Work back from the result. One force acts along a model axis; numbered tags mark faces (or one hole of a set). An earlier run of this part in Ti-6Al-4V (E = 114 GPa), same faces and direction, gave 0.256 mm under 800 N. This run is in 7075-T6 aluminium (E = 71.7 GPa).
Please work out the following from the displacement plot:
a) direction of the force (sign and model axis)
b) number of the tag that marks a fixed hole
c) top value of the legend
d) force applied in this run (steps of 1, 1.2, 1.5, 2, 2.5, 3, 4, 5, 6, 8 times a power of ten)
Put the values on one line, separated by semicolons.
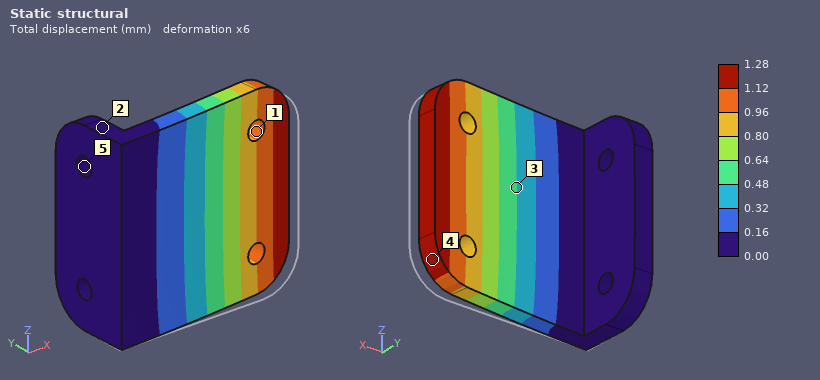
+Y; 5; 1.28 mm; 2.5 kN
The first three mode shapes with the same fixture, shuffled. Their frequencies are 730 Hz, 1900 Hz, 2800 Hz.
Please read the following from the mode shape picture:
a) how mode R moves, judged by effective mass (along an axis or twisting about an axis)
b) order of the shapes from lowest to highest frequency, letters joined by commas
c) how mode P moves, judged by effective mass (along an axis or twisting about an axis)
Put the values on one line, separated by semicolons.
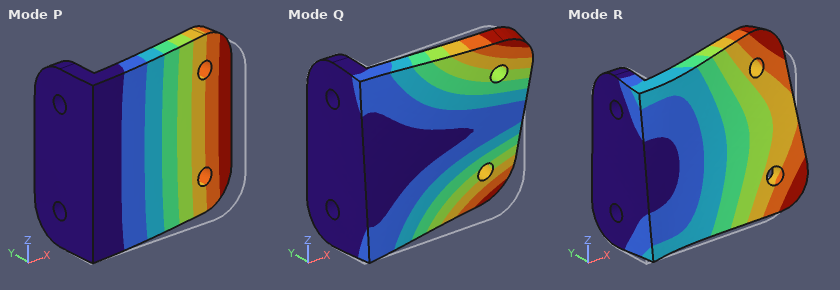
along Z; P, Q, R; along Y
